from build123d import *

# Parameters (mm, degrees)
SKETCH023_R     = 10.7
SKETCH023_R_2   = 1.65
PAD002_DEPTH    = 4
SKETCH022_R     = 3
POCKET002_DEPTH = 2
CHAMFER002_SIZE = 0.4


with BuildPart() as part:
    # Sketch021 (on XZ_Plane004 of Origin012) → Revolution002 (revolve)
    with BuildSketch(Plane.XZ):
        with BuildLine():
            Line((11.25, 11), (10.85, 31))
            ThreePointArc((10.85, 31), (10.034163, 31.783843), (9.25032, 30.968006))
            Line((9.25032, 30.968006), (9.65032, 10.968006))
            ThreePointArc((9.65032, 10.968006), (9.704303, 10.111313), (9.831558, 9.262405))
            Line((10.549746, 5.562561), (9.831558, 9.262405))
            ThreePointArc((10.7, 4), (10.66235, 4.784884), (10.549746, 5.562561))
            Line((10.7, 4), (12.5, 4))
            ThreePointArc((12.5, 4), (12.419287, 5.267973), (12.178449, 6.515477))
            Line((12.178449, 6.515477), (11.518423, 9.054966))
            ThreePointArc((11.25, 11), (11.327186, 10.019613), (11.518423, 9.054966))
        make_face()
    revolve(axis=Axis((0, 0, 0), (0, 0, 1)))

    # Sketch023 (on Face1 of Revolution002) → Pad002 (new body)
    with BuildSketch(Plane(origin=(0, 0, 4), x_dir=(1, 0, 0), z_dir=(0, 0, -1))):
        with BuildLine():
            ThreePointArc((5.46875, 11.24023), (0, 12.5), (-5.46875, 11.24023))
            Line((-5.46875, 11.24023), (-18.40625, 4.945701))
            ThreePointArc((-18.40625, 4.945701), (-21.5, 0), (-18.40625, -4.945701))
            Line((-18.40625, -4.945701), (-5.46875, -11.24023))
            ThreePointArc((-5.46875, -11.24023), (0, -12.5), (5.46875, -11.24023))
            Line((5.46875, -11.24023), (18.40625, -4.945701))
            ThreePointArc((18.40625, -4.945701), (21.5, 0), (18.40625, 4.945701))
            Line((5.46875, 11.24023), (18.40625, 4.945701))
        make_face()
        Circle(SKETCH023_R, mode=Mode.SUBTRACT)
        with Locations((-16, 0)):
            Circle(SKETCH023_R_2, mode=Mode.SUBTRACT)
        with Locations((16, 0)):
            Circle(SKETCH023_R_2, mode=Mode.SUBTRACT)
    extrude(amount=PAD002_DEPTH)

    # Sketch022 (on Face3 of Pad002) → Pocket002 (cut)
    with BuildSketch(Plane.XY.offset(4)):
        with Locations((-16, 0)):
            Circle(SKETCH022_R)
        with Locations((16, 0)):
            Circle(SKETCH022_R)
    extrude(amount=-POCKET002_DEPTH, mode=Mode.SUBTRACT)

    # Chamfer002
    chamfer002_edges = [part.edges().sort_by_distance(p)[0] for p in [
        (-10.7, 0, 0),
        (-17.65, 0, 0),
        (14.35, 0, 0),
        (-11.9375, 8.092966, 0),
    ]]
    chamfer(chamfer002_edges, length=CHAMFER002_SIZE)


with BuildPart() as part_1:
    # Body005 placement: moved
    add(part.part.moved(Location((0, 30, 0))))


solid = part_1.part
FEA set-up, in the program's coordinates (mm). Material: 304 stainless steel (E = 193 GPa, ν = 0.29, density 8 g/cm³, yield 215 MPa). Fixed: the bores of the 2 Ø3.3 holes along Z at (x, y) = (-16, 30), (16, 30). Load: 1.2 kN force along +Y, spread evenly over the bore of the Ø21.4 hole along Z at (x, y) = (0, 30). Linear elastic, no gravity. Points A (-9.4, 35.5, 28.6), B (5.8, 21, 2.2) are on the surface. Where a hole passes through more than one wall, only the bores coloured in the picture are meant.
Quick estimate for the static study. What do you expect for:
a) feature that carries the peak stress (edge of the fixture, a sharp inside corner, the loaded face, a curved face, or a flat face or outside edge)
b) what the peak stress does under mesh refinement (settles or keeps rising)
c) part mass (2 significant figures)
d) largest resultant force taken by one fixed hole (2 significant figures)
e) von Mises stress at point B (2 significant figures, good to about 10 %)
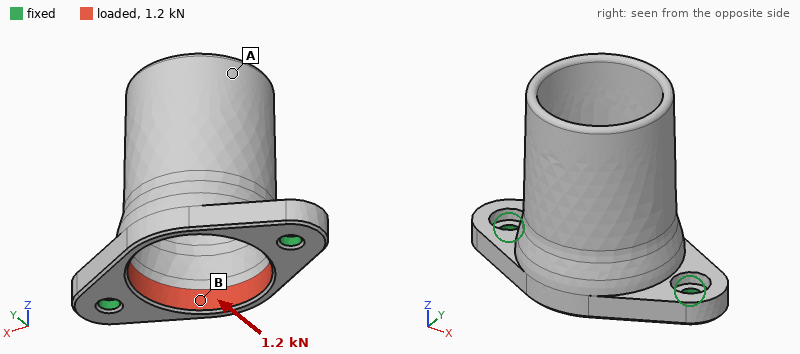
edge of the fixture
keeps rising
34 g
600 N
23 MPa
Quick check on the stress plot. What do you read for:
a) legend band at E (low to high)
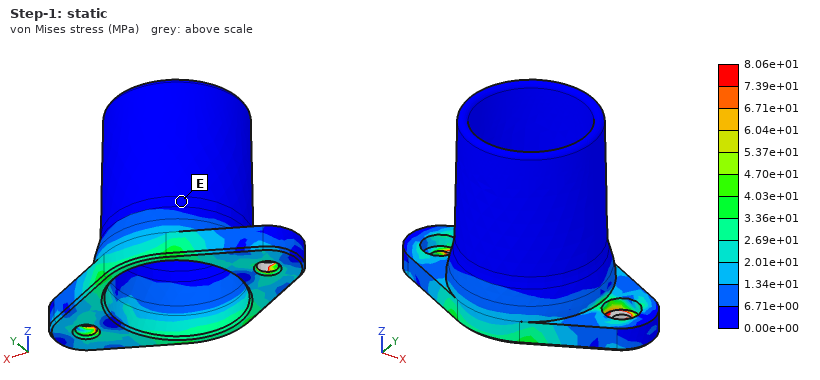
0.00e+00 to 6.71e+00 MPa
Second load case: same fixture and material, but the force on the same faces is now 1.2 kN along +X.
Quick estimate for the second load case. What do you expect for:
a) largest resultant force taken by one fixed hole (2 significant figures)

600 N
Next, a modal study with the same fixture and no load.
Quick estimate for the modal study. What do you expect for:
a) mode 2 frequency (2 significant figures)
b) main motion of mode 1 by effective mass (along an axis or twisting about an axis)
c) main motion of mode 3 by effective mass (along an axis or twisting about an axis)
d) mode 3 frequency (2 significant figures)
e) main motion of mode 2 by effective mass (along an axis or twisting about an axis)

9400 Hz
along Y
along X
11 kHz
along Z
